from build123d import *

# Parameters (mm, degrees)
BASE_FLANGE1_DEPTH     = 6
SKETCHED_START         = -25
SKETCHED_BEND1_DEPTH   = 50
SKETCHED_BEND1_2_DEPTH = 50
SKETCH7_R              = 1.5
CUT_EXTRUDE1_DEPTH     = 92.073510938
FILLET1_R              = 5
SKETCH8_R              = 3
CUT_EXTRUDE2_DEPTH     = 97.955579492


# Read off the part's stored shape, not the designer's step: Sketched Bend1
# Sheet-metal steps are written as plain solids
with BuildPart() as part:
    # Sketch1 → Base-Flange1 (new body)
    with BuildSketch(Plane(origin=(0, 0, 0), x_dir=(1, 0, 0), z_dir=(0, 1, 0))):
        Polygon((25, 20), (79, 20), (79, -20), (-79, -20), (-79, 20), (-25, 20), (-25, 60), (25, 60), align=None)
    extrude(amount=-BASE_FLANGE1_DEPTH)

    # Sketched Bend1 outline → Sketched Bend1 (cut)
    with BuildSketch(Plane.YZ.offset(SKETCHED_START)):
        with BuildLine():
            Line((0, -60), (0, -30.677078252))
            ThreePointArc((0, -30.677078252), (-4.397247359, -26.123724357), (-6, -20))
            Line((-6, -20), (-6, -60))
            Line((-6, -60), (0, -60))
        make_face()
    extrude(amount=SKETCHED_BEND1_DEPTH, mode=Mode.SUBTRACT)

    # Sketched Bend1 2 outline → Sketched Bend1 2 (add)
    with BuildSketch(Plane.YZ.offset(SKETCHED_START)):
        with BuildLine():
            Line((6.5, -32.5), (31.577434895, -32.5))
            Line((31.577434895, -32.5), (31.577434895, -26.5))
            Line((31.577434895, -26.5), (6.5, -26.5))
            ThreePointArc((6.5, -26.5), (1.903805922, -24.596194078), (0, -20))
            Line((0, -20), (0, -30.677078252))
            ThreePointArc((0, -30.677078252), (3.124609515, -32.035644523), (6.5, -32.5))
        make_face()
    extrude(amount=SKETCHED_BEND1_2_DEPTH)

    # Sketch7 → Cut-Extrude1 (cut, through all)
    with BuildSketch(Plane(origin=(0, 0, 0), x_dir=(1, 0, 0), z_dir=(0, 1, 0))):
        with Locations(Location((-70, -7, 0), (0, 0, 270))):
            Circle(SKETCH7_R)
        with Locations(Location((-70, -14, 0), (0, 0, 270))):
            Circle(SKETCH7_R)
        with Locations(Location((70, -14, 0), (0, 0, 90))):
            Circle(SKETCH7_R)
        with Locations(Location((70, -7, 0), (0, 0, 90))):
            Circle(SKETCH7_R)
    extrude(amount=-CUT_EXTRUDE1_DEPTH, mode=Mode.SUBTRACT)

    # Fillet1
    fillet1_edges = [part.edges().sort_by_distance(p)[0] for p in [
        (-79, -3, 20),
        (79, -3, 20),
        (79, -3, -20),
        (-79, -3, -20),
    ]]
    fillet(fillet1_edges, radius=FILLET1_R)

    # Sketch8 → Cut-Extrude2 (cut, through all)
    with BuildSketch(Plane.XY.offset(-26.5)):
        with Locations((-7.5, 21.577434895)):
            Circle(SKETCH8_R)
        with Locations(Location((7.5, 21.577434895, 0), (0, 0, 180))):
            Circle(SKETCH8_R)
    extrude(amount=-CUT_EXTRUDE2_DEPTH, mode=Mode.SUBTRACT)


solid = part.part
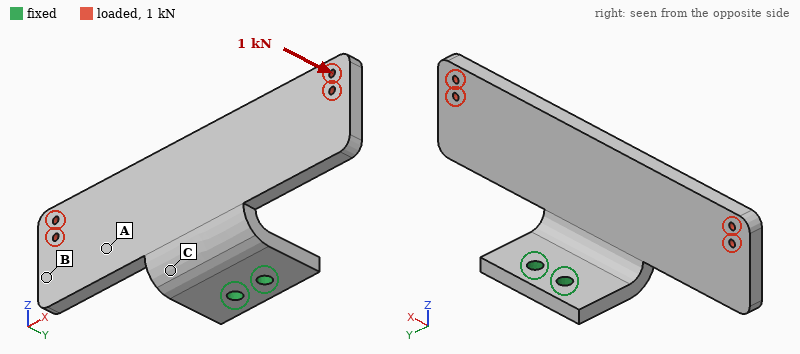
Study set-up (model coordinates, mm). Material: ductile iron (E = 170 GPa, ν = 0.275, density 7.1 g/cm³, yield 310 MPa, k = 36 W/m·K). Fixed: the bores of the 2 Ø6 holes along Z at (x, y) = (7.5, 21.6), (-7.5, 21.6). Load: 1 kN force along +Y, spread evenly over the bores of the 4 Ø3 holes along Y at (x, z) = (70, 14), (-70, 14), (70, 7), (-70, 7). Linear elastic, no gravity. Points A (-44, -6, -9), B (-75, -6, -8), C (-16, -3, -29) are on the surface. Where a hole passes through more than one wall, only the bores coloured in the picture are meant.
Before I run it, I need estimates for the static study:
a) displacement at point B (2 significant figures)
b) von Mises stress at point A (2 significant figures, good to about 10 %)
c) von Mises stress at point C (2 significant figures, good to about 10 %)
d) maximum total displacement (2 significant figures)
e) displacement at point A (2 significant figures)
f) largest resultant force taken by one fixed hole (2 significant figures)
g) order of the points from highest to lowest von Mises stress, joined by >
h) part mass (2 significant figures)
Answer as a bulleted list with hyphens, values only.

- 0.49 mm
- 57 MPa
- 97 MPa
- 0.79 mm
- 0.28 mm
- 540 N
- C > A > B
- 350 g
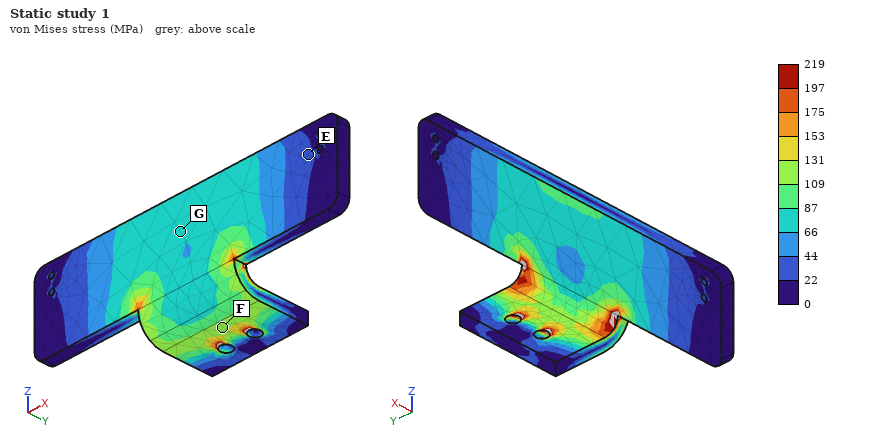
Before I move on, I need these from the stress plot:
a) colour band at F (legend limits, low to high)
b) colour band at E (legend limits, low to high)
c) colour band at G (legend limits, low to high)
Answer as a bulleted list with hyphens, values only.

- 109 to 131 MPa
- 22 to 44 MPa
- 66 to 87 MPa
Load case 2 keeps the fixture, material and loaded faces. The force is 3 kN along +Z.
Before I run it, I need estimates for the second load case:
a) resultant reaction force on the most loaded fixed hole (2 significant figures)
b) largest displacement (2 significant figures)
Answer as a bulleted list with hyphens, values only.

- 1.5 kN
- 0.33 mm
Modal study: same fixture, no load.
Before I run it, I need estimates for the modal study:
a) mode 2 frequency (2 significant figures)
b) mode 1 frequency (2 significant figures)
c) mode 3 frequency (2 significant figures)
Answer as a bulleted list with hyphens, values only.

- 620 Hz
- 600 Hz
- 850 Hz
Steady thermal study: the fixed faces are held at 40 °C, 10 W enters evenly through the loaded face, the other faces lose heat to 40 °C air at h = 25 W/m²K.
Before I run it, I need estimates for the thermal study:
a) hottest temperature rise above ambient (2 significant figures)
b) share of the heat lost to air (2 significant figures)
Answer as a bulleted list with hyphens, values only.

- 36 K
- 73 %
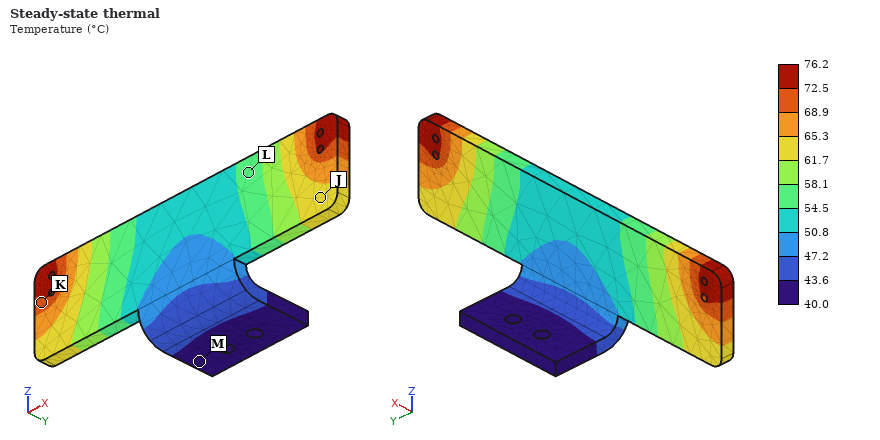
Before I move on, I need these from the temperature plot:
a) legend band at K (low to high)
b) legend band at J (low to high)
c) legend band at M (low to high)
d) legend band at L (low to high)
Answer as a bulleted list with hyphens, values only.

- 68.9 to 72.5 °C
- 61.7 to 65.3 °C
- 40.0 to 43.6 °C
- 54.5 to 58.1 °C
